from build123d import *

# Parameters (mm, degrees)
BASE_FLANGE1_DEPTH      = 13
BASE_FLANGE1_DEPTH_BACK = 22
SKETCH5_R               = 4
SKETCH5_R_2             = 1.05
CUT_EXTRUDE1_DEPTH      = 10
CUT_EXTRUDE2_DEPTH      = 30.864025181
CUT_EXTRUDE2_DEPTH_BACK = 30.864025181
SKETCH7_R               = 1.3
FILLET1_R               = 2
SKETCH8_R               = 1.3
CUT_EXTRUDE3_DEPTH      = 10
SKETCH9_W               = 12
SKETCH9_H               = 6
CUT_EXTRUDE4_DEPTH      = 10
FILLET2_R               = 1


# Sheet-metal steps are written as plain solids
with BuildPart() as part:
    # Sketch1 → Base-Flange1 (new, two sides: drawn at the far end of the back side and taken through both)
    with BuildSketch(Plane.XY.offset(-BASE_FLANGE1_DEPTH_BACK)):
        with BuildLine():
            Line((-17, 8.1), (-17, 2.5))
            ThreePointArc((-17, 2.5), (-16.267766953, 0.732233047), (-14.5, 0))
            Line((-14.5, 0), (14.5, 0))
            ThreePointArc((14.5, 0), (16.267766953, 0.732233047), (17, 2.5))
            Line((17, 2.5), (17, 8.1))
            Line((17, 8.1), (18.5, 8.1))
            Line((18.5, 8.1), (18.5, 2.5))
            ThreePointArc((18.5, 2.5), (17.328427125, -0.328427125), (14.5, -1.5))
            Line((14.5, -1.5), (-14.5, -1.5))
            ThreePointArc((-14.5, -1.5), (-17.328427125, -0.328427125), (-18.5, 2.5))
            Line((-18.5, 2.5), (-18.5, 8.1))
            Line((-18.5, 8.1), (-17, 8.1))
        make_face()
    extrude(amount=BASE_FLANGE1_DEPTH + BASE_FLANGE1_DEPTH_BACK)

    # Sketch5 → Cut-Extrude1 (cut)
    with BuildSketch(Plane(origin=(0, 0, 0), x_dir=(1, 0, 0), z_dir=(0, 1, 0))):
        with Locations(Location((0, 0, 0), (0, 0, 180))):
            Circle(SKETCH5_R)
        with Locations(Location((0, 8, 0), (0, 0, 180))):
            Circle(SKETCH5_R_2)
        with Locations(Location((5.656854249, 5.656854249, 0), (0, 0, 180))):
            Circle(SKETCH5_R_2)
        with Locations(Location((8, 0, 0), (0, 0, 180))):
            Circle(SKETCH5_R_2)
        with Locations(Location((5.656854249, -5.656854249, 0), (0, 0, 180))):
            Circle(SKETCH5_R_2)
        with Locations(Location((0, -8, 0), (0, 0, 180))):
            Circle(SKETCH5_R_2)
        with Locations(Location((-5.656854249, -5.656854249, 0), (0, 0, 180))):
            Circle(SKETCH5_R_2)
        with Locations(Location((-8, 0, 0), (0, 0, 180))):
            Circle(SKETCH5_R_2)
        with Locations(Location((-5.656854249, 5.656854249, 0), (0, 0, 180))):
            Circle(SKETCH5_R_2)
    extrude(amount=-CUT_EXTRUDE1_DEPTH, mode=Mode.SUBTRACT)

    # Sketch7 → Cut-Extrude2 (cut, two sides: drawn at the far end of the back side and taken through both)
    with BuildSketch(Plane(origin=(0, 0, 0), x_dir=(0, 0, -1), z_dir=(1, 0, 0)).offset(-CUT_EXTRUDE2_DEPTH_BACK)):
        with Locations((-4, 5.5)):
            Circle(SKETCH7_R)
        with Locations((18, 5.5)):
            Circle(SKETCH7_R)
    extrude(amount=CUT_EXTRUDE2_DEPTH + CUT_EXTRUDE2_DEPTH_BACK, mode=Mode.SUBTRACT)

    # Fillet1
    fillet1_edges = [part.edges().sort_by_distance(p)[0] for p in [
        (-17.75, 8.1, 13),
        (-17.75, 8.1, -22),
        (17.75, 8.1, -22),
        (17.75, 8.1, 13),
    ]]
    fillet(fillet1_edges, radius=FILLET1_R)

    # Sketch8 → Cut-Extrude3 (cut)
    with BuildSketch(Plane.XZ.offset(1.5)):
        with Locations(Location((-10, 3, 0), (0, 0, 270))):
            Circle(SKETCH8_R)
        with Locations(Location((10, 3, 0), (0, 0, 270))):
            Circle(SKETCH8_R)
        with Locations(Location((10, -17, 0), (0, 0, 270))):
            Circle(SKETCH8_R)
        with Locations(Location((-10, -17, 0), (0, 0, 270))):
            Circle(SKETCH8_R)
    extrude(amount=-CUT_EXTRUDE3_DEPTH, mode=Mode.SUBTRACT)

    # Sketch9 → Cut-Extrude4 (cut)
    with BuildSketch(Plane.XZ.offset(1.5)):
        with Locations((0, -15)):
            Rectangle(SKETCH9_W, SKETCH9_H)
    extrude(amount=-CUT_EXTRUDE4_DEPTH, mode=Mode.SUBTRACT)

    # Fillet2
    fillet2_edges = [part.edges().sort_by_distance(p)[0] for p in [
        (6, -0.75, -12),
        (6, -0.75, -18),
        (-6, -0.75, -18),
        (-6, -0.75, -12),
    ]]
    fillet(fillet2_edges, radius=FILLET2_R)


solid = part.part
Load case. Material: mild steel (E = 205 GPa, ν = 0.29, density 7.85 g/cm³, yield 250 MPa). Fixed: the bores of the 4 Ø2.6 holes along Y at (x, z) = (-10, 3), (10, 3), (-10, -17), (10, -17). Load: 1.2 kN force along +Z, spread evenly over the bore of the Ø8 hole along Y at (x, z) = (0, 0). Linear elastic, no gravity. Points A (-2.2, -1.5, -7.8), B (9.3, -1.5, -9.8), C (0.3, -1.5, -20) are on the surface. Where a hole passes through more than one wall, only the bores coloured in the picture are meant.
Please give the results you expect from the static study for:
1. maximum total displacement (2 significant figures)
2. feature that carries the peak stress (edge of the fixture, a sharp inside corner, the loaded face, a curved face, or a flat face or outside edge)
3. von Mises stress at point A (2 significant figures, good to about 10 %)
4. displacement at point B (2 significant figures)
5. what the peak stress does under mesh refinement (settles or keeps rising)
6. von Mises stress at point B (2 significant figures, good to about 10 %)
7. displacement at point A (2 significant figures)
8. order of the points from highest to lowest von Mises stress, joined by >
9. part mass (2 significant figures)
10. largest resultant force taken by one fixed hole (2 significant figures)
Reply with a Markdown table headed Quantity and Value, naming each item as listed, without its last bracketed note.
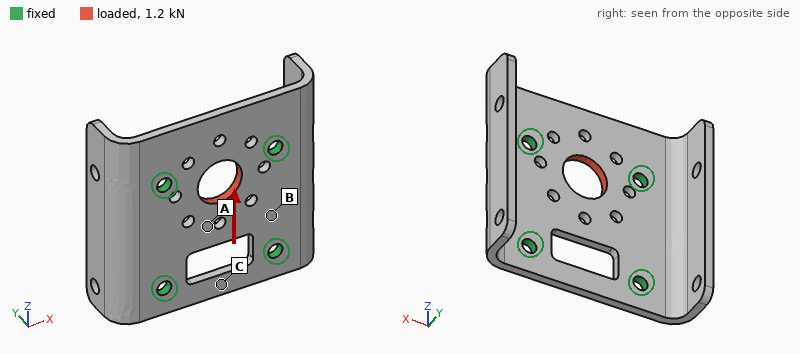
| Quantity | Value |
|---|---|
| maximum total displacement | 3.0 µm |
| feature that carries the peak stress | edge of the fixture |
| von Mises stress at point A | 20 MPa |
| displacement at point B | 0.57 µm |
| what the peak stress does under mesh refinement | keeps rising |
| von Mises stress at point B | 13 MPa |
| displacement at point A | 1.9 µm |
| order of the points from highest to lowest von Mises stress, joined by > | A > B > C |
| part mass | 18 g |
| largest resultant force taken by one fixed hole | 430 N |
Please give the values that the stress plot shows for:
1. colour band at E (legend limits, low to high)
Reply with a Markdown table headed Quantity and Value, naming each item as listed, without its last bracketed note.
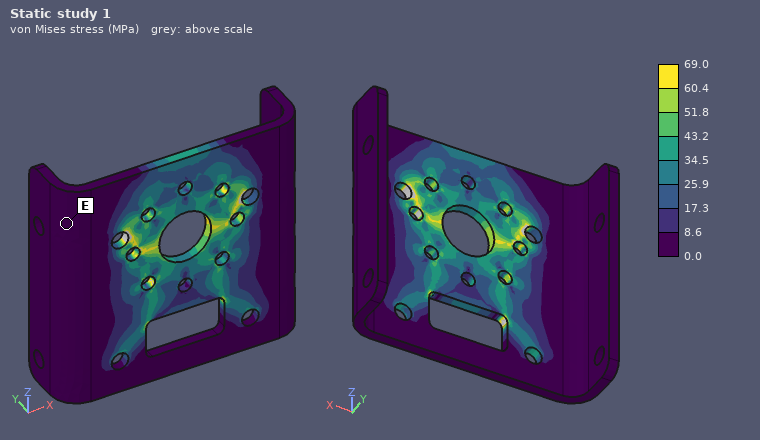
| Quantity | Value |
|---|---|
| colour band at E | 0.0 to 8.6 MPa |
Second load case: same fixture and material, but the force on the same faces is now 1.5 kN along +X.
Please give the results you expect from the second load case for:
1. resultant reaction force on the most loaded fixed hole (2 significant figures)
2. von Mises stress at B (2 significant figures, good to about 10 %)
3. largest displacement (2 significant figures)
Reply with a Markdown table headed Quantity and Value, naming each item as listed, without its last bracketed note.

| Quantity | Value |
|---|---|
| resultant reaction force on the most loaded fixed hole | 610 N |
| von Mises stress at B | 11 MPa |
| largest displacement | 2.7 µm |
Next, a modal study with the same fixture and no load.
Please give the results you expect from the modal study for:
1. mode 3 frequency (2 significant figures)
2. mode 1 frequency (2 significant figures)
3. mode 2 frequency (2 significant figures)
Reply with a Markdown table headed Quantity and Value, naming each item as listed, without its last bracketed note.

| Quantity | Value |
|---|---|
| mode 3 frequency | 8700 Hz |
| mode 1 frequency | 6300 Hz |
| mode 2 frequency | 6400 Hz |
